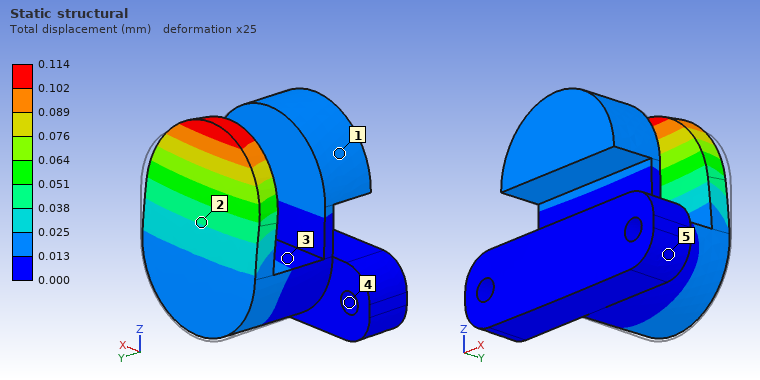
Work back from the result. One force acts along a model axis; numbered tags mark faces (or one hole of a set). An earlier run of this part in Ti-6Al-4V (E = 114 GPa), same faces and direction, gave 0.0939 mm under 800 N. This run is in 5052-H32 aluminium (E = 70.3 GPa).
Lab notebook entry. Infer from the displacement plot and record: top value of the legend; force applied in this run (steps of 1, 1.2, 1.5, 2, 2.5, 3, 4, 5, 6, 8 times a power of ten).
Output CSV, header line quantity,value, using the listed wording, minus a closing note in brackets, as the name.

quantity,value
top value of the legend,0.114 mm
force applied in this run,600 N
